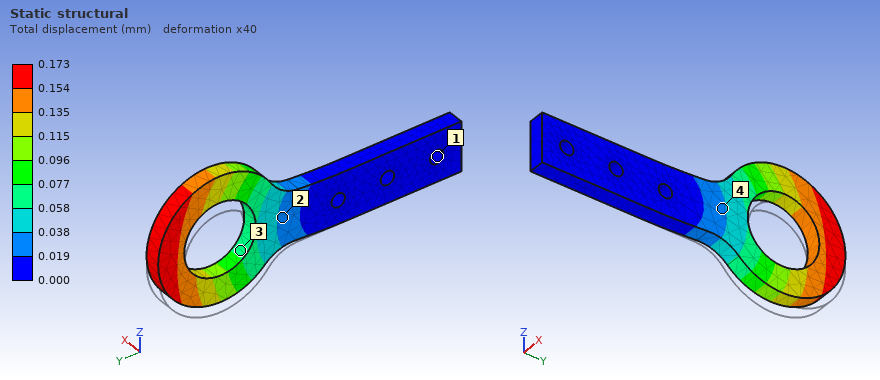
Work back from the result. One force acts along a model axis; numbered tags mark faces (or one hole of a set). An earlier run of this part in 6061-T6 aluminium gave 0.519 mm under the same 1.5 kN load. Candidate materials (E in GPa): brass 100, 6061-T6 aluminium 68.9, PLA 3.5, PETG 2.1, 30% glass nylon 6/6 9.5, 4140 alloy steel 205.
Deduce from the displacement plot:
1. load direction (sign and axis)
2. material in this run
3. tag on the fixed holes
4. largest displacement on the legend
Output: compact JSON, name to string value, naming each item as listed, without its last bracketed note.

{"load direction": "+Z", "material in this run": "4140 alloy steel", "tag on the fixed holes": "1", "largest displacement on the legend": "0.173 mm"}
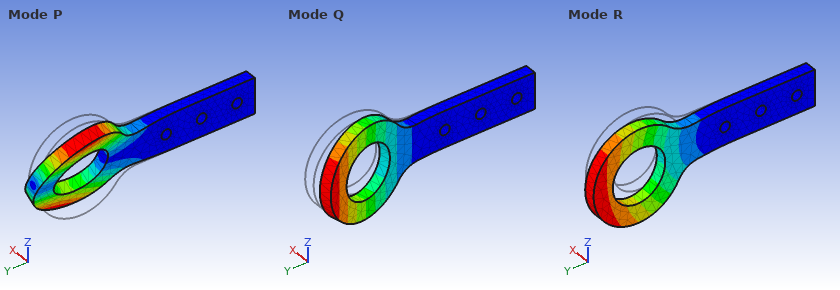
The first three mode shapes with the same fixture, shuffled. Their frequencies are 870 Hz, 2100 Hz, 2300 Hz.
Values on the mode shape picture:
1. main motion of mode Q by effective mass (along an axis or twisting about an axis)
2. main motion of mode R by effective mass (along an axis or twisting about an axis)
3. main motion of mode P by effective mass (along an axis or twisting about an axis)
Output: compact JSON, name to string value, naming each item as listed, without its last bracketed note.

{"main motion of mode Q by effective mass": "along X", "main motion of mode R by effective mass": "along Z", "main motion of mode P by effective mass": "twisting about Y"}
